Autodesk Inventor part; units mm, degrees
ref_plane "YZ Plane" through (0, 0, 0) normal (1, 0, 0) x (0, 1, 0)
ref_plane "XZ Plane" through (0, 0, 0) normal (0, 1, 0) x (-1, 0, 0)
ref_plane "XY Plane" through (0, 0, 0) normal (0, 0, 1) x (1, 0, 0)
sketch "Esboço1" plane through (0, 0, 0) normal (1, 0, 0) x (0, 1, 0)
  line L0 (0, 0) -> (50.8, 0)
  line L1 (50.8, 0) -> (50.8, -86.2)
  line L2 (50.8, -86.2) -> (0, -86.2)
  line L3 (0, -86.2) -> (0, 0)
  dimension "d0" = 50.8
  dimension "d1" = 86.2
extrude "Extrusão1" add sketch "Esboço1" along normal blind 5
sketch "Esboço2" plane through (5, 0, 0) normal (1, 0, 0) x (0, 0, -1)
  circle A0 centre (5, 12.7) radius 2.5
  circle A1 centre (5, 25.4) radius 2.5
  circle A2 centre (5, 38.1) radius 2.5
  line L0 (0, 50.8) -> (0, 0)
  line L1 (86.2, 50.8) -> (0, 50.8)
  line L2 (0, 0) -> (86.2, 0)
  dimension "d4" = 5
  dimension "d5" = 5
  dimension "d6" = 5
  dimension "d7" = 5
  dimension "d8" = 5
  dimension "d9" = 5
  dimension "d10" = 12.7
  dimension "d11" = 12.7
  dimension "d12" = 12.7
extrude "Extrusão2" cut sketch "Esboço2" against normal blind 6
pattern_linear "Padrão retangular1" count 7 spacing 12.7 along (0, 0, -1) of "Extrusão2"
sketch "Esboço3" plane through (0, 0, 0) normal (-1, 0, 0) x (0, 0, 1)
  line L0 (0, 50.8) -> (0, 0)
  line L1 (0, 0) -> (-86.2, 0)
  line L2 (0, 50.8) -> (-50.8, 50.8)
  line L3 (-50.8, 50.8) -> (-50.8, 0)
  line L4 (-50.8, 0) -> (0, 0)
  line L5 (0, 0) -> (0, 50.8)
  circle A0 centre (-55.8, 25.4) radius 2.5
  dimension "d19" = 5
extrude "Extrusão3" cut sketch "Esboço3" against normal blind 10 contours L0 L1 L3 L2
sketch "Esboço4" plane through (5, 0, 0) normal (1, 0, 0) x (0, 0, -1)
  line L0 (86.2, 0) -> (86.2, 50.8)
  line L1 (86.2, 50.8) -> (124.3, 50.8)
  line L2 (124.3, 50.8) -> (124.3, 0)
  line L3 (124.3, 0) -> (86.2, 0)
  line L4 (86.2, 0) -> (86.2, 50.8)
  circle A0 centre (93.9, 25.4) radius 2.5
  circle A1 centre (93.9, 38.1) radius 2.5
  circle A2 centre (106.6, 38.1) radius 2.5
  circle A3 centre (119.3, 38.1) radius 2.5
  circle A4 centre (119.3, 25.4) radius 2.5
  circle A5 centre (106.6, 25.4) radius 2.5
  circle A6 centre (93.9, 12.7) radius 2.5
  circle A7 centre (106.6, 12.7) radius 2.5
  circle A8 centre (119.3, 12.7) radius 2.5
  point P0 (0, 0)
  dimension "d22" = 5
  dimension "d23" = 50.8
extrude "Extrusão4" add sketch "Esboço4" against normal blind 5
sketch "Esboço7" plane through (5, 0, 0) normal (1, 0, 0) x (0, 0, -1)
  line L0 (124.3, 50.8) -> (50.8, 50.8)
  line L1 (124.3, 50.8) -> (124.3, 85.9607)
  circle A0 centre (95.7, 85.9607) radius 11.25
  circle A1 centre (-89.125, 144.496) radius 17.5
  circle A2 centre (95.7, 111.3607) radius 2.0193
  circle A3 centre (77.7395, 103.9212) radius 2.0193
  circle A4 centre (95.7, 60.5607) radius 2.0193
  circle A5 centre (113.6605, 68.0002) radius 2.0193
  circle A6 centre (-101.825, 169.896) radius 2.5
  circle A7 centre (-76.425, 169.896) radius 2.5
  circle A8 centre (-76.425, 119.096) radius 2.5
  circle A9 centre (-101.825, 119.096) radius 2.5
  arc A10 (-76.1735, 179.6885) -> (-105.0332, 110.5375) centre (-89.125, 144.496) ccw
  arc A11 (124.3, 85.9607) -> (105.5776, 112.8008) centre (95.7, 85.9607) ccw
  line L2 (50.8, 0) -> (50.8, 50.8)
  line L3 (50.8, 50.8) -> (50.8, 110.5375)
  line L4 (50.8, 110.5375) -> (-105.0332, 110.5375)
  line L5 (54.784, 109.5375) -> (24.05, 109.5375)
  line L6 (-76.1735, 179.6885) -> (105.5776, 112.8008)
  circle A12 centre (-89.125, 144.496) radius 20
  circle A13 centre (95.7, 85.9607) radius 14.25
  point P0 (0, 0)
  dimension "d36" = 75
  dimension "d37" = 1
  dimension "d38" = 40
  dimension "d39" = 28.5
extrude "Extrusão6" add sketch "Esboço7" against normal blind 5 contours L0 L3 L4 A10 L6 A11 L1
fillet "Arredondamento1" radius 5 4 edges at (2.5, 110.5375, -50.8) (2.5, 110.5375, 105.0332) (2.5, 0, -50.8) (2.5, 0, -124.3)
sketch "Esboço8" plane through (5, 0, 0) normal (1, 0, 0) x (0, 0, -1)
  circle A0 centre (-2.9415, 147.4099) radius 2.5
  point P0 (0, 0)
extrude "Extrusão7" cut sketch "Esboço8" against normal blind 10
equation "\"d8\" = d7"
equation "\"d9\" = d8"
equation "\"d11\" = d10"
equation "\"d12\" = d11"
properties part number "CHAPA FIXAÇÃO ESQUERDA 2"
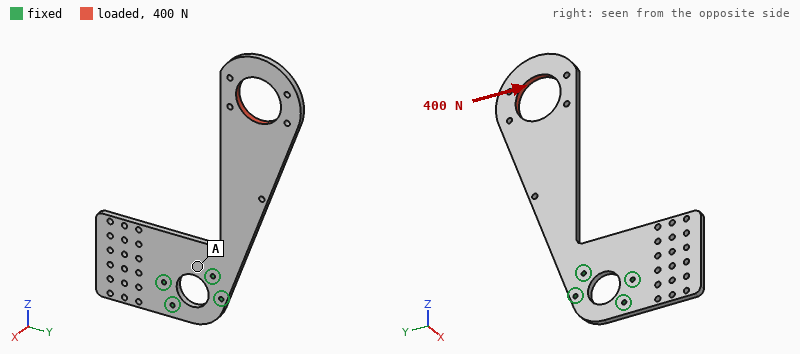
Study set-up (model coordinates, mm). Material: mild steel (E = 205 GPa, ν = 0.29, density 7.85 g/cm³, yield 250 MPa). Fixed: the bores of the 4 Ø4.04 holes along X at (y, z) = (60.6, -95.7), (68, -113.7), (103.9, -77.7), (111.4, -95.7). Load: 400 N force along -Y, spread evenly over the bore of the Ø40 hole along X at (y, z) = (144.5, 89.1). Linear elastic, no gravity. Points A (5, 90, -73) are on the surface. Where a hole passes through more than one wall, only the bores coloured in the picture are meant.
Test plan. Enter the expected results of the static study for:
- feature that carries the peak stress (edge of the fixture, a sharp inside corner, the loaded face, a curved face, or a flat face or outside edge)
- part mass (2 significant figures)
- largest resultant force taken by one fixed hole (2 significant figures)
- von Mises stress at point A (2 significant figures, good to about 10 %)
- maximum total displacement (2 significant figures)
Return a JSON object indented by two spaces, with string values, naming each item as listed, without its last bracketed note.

{
  "feature that carries the peak stress": "a curved face",
  "part mass": "600 g",
  "largest resultant force taken by one fixed hole": "1.4 kN",
  "von Mises stress at point A": "14 MPa",
  "maximum total displacement": "0.43 mm"
}
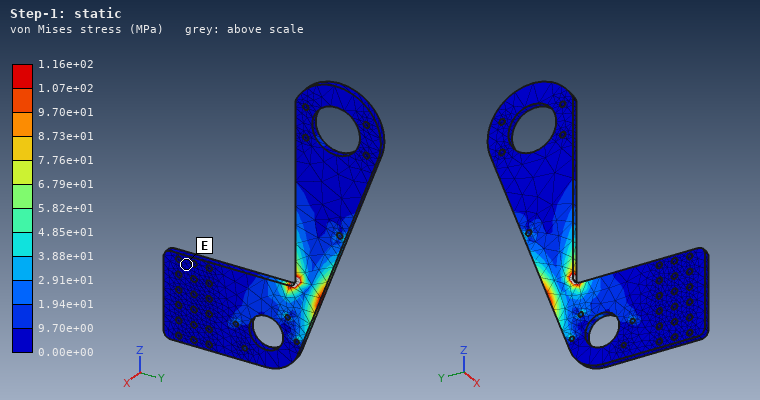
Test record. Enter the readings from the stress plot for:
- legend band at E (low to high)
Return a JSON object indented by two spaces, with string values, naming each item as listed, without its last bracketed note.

{
  "legend band at E": "0.00e+00 to 9.70e+00 MPa"
}
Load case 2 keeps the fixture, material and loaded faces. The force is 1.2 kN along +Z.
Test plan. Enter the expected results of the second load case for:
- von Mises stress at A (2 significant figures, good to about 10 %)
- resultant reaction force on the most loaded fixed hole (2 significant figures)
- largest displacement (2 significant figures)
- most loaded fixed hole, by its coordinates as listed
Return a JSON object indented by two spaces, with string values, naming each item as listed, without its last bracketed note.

{
  "von Mises stress at A": "8.9 MPa",
  "resultant reaction force on the most loaded fixed hole": "1.3 kN",
  "largest displacement": "0.24 mm",
  "most loaded fixed hole, by its coordinates as listed": "(111.4, -95.7)"
}
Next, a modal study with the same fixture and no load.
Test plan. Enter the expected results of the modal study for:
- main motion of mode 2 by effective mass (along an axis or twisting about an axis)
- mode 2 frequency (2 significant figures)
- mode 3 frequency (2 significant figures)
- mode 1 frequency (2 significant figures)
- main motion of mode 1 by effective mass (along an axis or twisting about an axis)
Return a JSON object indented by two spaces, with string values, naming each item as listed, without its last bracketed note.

{
  "main motion of mode 2 by effective mass": "along Y",
  "mode 2 frequency": "420 Hz",
  "mode 3 frequency": "470 Hz",
  "mode 1 frequency": "80 Hz",
  "main motion of mode 1 by effective mass": "along X"
}
